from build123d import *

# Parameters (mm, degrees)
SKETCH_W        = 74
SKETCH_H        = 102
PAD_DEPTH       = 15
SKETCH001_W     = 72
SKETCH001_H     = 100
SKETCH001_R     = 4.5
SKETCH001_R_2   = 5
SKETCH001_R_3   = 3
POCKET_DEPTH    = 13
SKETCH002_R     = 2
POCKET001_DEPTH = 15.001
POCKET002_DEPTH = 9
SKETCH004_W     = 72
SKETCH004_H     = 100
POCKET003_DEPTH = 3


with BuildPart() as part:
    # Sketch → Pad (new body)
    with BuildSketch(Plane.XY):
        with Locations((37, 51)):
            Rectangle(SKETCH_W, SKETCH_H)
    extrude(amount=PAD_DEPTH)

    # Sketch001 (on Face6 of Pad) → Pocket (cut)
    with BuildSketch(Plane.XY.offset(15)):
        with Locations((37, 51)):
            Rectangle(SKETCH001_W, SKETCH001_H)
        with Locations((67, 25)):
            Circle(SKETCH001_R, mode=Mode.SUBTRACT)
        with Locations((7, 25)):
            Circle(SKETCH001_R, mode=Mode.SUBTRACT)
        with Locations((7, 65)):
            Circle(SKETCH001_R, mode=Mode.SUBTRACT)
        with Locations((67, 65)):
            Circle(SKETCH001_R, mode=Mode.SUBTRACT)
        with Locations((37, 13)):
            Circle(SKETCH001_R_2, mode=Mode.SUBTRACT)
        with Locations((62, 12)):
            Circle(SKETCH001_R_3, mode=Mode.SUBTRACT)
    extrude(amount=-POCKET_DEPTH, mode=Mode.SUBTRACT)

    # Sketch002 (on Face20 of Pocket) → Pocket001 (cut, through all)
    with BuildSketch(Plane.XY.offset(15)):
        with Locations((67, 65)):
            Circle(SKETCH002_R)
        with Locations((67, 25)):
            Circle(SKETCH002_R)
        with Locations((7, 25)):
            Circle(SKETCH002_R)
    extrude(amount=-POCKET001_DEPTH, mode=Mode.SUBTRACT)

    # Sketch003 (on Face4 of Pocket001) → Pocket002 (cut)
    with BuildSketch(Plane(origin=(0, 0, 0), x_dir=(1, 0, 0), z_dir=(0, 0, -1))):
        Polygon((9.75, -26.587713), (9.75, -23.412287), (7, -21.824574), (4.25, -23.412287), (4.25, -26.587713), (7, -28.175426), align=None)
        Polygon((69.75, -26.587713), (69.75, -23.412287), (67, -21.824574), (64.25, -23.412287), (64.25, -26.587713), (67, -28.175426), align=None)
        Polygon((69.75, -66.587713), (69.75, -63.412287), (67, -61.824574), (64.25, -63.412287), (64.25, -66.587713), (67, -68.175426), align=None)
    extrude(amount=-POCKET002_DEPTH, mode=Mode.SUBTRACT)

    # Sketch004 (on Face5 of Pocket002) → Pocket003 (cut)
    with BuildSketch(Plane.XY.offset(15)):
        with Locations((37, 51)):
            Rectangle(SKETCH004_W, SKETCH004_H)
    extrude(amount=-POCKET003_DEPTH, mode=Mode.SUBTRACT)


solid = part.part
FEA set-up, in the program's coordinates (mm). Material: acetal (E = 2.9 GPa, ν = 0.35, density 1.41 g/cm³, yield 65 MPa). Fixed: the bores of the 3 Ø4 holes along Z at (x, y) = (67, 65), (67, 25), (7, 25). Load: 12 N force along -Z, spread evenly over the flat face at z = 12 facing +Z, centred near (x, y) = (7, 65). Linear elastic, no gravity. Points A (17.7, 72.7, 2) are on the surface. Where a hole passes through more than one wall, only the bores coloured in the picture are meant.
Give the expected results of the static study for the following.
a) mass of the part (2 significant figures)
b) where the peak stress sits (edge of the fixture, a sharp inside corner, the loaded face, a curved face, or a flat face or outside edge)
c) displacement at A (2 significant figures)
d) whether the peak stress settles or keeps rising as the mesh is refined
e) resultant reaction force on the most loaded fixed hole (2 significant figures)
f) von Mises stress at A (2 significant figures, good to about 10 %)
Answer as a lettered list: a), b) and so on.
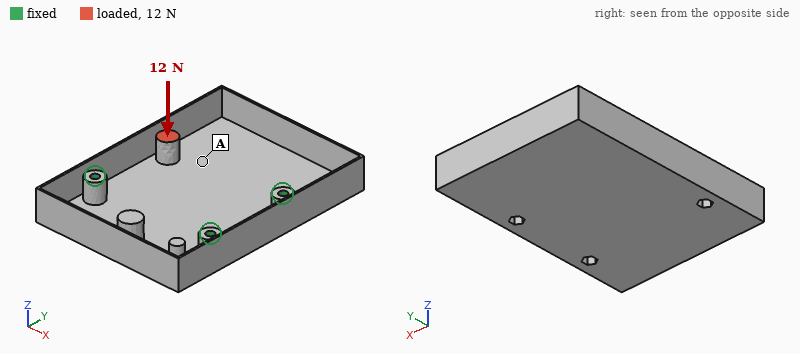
a) 32 g
b) edge of the fixture
c) 0.65 mm
d) keeps rising
e) 13 N
f) 0.90 MPa
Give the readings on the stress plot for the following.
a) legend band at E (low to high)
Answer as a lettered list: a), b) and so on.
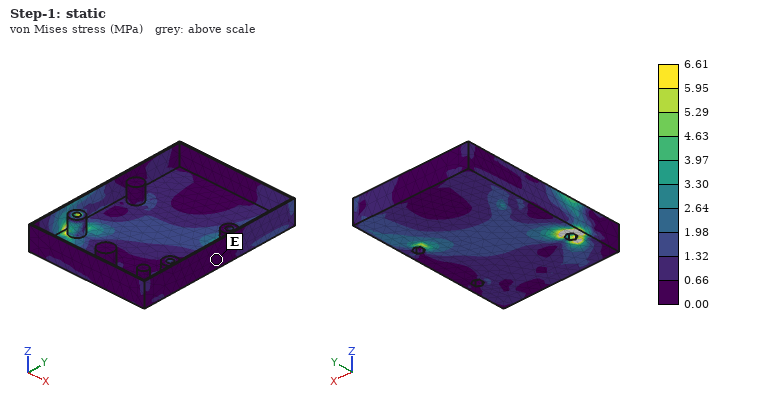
a) 0.00 to 0.66 MPa
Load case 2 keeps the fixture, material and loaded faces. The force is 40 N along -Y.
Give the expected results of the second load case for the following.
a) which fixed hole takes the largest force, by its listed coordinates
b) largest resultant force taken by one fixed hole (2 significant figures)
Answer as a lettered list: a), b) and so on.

a) (7, 25)
b) 39 N
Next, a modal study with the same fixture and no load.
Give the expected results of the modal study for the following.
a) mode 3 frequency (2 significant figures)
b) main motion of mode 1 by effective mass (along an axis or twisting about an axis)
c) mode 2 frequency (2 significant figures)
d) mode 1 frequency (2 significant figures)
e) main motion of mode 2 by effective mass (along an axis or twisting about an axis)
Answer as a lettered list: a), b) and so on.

a) 800 Hz
b) along Z
c) 680 Hz
d) 190 Hz
e) along Z
